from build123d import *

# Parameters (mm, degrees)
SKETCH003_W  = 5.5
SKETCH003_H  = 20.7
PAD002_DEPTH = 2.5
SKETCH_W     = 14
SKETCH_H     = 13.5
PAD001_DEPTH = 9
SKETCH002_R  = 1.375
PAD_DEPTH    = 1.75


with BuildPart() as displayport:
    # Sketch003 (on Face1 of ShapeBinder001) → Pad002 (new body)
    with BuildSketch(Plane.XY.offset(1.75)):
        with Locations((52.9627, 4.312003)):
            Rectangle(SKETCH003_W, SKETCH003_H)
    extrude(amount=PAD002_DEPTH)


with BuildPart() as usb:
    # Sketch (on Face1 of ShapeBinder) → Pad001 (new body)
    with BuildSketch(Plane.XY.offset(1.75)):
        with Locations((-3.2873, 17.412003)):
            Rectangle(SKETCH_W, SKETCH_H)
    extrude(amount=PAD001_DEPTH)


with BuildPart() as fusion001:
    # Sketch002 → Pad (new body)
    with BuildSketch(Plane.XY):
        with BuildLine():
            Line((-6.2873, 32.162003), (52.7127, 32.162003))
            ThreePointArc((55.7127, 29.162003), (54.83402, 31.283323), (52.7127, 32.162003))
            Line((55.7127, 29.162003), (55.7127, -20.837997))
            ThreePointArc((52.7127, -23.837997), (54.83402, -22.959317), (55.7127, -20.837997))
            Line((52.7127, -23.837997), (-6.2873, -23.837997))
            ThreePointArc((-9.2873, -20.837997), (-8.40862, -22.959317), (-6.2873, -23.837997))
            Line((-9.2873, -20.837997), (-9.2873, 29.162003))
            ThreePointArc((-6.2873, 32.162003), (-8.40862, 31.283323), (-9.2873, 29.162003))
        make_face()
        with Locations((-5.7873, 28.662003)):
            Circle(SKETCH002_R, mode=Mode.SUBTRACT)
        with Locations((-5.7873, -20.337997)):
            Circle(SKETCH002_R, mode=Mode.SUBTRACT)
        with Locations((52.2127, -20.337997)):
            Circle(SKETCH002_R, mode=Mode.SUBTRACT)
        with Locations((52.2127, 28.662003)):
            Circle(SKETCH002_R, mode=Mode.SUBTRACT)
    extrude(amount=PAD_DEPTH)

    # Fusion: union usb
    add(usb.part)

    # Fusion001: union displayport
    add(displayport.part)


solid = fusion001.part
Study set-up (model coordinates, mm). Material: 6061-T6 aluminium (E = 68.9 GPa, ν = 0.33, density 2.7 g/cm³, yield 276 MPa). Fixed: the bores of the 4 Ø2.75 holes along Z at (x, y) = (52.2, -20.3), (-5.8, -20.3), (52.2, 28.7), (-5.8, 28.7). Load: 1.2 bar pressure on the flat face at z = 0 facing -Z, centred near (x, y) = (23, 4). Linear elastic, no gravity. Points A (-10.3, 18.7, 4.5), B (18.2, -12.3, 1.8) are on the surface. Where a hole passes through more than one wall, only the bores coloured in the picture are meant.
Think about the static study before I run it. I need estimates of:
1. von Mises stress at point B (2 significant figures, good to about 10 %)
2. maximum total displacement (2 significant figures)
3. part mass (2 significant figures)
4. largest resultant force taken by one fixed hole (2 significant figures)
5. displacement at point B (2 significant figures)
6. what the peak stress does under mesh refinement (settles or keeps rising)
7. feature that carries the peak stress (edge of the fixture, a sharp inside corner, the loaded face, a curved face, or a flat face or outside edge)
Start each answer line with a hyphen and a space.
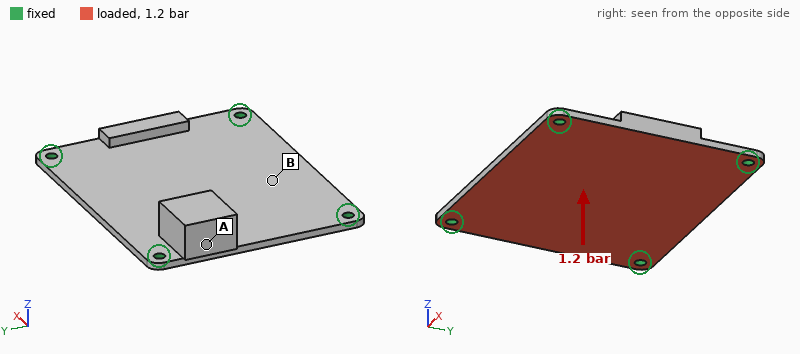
- 36 MPa
- 0.21 mm
- 22 g
- 110 N
- 0.18 mm
- keeps rising
- edge of the fixture
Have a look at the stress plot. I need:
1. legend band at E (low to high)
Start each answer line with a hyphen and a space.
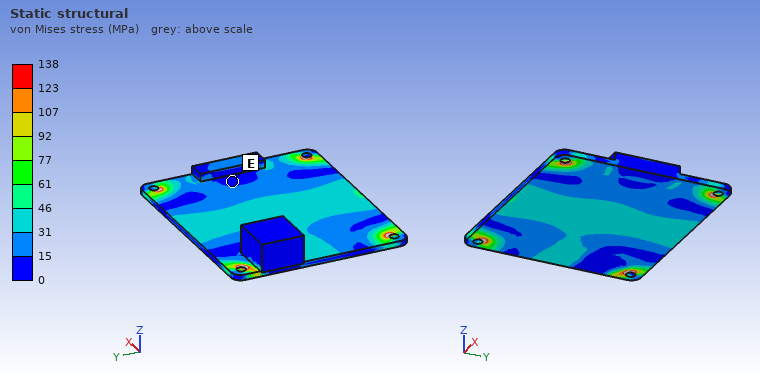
- 0 to 15 MPa
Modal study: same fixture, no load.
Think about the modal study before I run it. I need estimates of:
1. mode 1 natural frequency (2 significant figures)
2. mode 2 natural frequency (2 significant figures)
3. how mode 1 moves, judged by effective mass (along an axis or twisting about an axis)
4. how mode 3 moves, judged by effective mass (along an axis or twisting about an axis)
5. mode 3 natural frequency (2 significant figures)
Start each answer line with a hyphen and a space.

- 2000 Hz
- 3200 Hz
- along Z
- twisting about X
- 3400 Hz
